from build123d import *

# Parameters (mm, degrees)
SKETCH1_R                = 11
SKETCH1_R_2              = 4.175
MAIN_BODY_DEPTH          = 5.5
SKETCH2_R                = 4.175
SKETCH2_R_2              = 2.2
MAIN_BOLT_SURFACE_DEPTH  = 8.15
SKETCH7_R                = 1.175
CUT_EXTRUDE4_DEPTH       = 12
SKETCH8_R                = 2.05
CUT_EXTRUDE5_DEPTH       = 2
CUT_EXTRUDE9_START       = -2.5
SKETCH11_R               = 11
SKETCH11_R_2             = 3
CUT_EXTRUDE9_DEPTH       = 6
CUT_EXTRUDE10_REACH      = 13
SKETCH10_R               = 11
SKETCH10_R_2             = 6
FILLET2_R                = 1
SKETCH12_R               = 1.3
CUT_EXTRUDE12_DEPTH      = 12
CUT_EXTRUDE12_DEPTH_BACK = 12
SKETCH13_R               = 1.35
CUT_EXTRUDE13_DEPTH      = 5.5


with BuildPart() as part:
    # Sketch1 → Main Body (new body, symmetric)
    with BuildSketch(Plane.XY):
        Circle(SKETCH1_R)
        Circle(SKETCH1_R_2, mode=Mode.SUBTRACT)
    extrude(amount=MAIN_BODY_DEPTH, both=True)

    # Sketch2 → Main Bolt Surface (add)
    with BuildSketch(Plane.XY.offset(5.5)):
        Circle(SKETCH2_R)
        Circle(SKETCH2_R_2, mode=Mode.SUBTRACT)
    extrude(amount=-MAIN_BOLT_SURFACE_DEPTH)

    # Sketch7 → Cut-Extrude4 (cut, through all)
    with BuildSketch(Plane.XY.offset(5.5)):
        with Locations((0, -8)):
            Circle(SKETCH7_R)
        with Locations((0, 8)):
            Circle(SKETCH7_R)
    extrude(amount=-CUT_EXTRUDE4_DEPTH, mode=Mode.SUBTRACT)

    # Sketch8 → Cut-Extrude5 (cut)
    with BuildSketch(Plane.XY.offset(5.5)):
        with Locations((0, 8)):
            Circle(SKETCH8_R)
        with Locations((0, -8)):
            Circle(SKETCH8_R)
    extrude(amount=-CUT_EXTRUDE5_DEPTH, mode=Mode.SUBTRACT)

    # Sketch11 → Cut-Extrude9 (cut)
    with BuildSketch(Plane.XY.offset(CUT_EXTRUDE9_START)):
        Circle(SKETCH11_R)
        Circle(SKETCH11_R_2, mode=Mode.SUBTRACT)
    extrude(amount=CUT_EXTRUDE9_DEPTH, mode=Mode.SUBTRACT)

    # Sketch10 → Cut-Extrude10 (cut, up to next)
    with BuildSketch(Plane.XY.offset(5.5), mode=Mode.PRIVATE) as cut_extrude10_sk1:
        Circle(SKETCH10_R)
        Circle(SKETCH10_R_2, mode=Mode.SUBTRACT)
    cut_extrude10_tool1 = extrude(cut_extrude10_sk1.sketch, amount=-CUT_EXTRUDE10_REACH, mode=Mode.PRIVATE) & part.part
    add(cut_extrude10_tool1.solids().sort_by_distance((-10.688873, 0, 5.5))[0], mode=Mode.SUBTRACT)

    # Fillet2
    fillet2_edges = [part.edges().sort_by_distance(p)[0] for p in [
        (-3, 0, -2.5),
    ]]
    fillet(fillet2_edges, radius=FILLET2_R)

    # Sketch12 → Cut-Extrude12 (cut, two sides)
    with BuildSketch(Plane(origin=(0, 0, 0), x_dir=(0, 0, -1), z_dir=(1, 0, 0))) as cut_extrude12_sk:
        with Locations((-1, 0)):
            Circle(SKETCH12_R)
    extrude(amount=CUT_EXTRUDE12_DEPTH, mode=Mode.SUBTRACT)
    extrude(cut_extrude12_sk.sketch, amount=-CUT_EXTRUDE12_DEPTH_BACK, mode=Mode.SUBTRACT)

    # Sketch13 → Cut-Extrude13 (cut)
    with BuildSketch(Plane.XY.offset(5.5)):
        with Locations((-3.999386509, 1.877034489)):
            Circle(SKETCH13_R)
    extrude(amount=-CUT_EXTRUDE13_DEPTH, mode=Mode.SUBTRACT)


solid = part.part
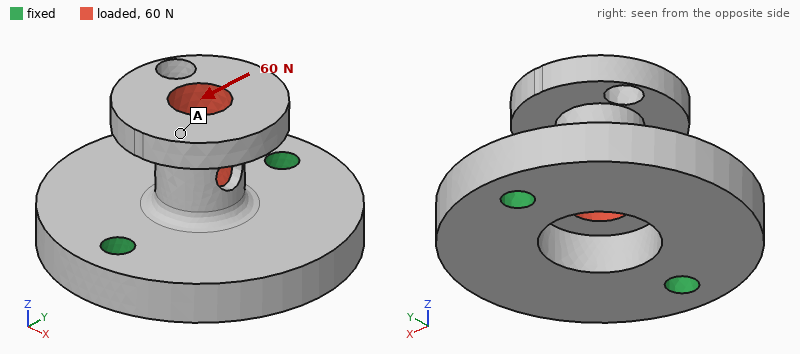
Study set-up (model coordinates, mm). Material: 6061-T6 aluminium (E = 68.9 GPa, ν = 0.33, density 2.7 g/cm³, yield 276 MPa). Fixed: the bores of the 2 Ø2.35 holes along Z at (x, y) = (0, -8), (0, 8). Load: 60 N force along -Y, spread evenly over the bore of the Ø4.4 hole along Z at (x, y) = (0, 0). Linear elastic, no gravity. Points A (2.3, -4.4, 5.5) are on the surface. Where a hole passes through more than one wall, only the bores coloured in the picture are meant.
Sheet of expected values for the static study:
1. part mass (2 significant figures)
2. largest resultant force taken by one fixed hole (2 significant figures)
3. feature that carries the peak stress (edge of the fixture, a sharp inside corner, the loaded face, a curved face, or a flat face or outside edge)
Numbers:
3.3 g
40 N
a curved face
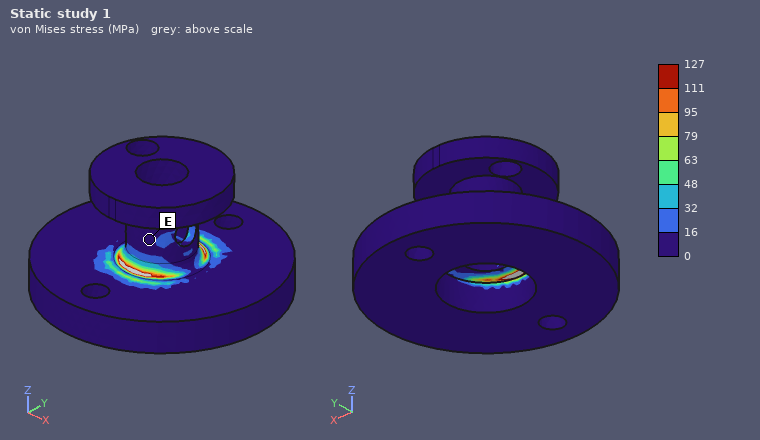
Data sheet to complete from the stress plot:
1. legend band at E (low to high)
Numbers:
0 to 16 MPa
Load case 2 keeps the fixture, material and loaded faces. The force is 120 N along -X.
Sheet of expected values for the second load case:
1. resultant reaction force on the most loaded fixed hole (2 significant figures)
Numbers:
60 N
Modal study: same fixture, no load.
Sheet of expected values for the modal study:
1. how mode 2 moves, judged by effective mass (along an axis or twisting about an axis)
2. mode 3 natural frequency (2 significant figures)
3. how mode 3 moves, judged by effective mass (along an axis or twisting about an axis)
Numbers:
along Y
20 kHz
along Z
